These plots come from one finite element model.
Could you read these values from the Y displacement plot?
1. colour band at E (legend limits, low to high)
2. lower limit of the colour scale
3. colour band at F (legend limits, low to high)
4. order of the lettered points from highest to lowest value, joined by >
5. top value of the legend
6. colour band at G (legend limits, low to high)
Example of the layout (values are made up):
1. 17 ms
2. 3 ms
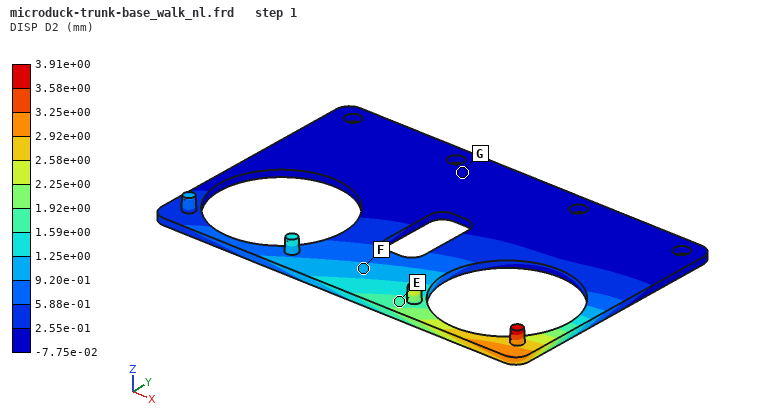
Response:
1. 1.59e+00 to 1.92e+00 mm
2. -7.75e-02 mm
3. 9.20e-01 to 1.25e+00 mm
4. E > F > G
5. 3.91e+00 mm
6. -7.75e-02 to 2.55e-01 mm
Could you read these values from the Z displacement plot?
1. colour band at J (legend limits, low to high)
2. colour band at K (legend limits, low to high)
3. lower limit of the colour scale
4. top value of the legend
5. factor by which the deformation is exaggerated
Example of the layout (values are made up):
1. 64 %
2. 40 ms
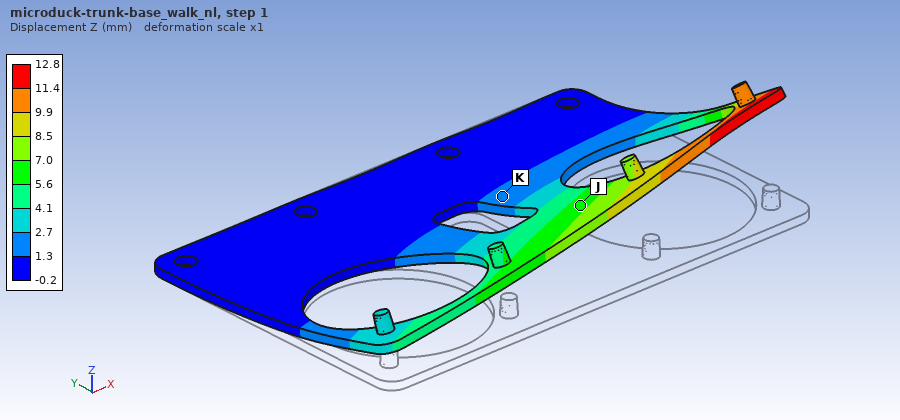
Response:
1. 5.6 to 7.0 mm
2. 1.3 to 2.7 mm
3. -0.2 mm
4. 12.8 mm
5. 1
